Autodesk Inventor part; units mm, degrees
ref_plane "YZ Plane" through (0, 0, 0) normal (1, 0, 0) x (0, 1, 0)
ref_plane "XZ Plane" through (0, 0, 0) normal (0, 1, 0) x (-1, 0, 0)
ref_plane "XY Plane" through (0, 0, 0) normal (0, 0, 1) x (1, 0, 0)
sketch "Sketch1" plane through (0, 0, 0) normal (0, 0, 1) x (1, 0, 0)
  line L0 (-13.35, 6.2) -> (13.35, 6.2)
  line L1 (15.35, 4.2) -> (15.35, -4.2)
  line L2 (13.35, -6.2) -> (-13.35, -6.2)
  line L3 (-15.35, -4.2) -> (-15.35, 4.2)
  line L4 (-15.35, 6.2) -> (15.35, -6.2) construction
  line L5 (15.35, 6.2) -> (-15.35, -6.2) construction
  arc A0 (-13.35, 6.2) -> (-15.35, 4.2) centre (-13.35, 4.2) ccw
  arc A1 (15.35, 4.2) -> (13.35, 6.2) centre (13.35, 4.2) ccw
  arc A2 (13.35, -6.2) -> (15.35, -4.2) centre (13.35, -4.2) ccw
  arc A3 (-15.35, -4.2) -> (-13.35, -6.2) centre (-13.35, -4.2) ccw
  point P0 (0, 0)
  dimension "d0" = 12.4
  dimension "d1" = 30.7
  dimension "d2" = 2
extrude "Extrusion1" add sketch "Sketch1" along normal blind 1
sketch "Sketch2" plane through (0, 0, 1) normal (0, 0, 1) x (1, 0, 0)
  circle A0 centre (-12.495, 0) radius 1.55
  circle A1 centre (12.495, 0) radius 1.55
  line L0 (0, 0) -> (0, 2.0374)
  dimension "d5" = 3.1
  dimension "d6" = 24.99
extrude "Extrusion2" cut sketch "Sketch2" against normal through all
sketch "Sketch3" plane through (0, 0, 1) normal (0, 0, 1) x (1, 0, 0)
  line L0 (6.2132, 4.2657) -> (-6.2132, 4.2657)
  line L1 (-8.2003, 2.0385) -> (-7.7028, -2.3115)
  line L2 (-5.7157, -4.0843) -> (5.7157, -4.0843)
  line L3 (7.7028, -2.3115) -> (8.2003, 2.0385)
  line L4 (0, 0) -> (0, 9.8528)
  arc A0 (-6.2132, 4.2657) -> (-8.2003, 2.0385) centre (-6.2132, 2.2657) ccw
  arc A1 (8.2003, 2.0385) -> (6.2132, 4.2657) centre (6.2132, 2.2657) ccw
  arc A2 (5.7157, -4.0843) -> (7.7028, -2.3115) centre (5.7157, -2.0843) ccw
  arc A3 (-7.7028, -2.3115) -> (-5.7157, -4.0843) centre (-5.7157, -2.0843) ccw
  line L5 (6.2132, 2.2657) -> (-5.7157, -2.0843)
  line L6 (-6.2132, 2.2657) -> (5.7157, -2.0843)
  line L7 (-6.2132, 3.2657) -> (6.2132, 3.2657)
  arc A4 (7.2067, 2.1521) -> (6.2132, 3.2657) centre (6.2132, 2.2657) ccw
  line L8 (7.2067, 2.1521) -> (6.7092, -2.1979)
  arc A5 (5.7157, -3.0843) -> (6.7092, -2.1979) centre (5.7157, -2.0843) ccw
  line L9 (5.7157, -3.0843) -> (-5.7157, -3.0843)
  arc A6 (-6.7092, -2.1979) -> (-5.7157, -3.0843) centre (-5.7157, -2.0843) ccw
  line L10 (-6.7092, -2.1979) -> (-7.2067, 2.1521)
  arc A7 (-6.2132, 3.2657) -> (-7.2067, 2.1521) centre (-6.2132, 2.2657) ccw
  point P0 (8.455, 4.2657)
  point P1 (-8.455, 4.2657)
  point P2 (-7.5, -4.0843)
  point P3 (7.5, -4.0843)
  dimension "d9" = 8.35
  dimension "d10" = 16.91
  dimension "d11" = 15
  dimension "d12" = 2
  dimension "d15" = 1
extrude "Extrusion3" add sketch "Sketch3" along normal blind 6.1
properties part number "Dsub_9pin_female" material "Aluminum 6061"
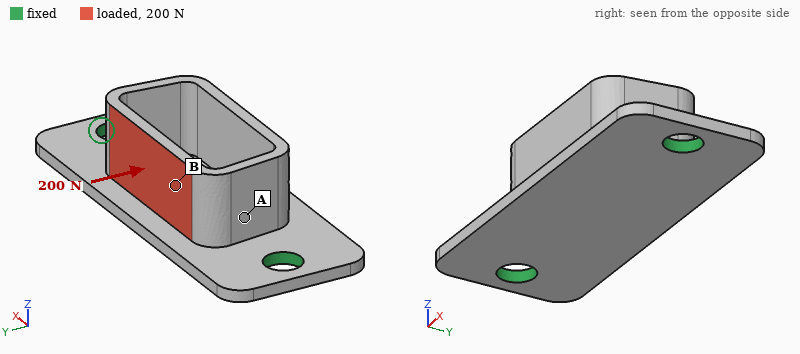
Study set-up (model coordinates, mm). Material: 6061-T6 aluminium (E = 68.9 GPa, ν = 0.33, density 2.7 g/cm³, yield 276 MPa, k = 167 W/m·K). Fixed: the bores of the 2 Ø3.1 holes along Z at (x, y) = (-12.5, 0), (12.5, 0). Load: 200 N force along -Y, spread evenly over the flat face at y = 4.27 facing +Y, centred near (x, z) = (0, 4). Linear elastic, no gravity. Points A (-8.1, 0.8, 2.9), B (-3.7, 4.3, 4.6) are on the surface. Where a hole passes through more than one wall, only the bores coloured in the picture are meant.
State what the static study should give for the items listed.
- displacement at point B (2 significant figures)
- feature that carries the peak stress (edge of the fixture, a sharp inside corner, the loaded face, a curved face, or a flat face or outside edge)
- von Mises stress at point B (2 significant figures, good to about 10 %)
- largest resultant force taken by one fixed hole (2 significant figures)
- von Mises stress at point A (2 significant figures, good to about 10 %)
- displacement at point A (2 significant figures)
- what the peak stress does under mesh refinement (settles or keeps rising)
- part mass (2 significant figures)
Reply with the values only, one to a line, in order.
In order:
0.080 mm
edge of the fixture
78 MPa
100 N
26 MPa
0.027 mm
keeps rising
1.7 g
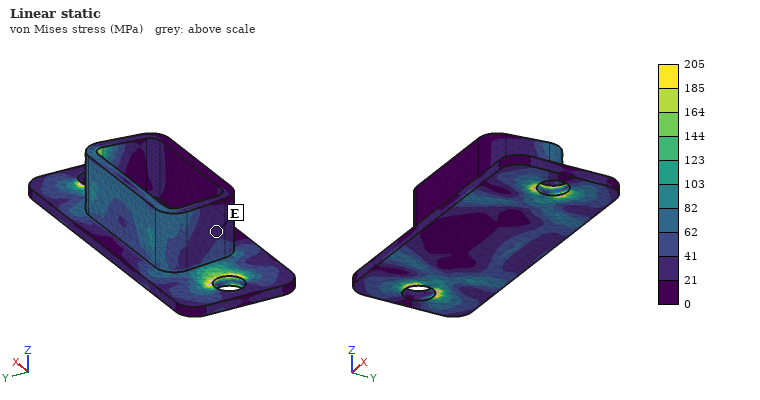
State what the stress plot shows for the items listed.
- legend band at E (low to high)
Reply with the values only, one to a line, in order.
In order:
21 to 41 MPa
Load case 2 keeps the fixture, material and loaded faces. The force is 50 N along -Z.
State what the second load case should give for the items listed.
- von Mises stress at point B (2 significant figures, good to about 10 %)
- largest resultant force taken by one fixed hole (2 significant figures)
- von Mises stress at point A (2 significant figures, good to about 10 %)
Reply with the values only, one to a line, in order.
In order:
10 MPa
29 N
8.2 MPa
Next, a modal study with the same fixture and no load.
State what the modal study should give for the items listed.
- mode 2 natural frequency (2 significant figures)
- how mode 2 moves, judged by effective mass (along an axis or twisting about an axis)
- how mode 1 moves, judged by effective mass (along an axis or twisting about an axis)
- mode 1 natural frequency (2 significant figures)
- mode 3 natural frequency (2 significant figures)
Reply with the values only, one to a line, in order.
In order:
15 kHz
along Z
along Y
8400 Hz
20 kHz
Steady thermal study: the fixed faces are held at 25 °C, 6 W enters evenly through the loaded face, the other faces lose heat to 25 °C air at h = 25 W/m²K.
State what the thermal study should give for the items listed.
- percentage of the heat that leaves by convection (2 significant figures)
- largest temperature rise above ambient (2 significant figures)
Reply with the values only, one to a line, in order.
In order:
4.0 %
19 K
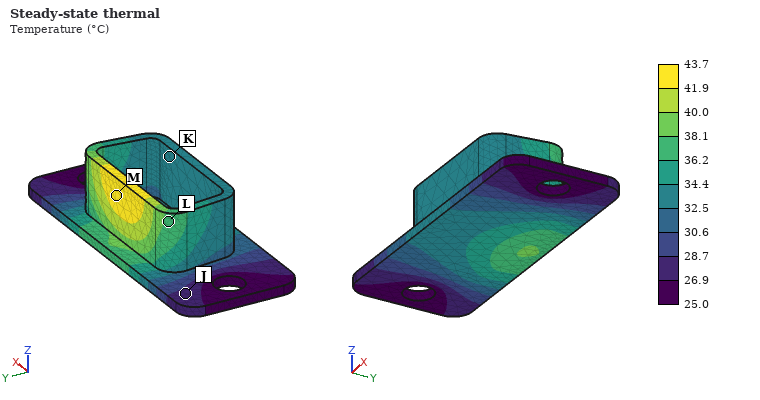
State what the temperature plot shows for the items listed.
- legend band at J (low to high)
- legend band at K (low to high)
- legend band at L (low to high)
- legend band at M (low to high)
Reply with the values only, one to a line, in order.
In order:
26.9 to 28.7 °C
32.5 to 34.4 °C
36.2 to 38.1 °C
41.9 to 43.7 °C
